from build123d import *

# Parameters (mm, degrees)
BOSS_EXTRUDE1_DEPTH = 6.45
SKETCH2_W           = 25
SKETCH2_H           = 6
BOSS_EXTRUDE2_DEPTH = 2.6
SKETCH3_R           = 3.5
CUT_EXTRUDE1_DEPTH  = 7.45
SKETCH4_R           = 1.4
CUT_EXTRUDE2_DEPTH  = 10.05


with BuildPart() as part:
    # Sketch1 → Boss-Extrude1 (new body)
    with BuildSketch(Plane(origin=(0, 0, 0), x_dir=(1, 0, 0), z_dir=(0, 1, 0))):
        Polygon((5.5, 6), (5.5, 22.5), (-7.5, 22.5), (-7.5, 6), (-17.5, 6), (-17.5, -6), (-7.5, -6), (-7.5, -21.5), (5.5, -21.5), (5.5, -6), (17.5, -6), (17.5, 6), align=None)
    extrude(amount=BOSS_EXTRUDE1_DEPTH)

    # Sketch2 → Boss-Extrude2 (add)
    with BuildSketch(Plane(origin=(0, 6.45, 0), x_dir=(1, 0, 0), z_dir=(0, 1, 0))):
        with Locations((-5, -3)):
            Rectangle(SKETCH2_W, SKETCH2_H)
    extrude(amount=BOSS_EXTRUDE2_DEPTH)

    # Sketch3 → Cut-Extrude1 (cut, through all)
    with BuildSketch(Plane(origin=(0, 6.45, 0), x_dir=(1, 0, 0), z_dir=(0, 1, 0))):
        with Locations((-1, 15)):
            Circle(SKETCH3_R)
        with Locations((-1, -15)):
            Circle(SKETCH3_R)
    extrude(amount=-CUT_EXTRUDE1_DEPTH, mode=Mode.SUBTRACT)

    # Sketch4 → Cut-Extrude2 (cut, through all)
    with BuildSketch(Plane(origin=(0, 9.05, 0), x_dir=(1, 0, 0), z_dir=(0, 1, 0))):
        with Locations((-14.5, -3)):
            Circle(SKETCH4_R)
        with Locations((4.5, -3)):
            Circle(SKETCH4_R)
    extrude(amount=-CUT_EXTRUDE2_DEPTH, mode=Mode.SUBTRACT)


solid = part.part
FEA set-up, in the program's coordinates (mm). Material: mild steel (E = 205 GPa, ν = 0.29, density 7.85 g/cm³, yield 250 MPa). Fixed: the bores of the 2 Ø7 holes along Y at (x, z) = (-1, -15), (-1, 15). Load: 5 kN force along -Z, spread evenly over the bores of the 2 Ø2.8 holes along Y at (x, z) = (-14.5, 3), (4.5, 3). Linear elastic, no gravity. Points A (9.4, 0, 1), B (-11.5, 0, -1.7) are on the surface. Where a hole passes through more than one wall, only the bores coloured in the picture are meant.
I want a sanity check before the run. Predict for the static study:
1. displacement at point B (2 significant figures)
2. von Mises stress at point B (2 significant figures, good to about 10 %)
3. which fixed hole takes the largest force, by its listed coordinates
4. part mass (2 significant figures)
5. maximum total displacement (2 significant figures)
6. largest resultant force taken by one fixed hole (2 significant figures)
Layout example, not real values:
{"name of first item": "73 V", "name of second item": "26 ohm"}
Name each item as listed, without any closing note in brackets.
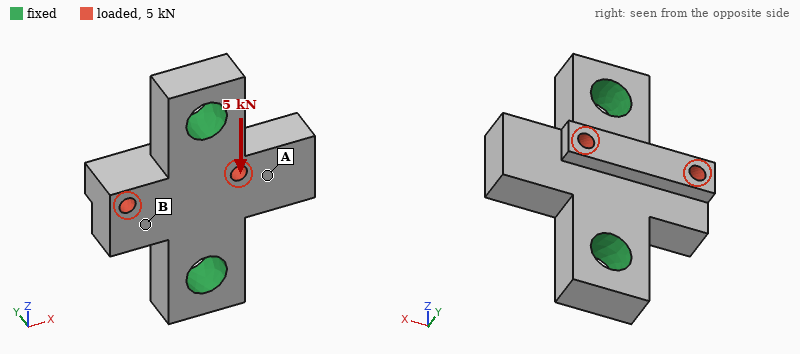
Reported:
{"displacement at point B": "5.0 µm", "von Mises stress at point B": "44 MPa", "which fixed hole takes the largest force, by its listed coordinates": "(-1, 15)", "part mass": "41 g", "maximum total displacement": "15 µm", "largest resultant force taken by one fixed hole": "2.9 kN"}
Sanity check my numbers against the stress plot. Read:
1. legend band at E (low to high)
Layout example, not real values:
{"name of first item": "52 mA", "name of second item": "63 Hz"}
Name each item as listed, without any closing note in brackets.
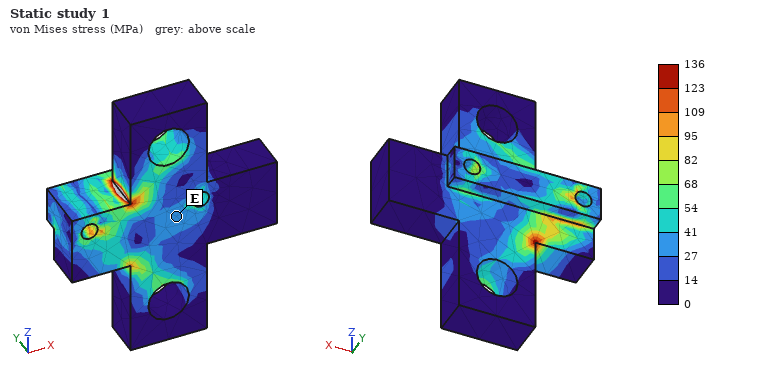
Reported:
{"legend band at E": "27 to 41 MPa"}
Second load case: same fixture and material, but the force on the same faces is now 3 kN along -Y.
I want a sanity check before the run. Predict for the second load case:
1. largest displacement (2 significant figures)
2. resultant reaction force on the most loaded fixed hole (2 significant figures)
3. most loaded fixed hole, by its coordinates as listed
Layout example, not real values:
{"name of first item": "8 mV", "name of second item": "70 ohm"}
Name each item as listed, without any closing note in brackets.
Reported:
{"largest displacement": "32 µm", "resultant reaction force on the most loaded fixed hole": "2.0 kN", "most loaded fixed hole, by its coordinates as listed": "(-1, 15)"}
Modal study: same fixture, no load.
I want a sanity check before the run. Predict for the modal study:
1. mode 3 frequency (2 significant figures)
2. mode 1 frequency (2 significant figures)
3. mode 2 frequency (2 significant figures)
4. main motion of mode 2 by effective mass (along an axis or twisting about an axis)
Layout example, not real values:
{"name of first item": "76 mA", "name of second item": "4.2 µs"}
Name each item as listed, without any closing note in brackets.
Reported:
{"mode 3 frequency": "29 kHz", "mode 1 frequency": "12 kHz", "mode 2 frequency": "18 kHz", "main motion of mode 2 by effective mass": "along Y"}
